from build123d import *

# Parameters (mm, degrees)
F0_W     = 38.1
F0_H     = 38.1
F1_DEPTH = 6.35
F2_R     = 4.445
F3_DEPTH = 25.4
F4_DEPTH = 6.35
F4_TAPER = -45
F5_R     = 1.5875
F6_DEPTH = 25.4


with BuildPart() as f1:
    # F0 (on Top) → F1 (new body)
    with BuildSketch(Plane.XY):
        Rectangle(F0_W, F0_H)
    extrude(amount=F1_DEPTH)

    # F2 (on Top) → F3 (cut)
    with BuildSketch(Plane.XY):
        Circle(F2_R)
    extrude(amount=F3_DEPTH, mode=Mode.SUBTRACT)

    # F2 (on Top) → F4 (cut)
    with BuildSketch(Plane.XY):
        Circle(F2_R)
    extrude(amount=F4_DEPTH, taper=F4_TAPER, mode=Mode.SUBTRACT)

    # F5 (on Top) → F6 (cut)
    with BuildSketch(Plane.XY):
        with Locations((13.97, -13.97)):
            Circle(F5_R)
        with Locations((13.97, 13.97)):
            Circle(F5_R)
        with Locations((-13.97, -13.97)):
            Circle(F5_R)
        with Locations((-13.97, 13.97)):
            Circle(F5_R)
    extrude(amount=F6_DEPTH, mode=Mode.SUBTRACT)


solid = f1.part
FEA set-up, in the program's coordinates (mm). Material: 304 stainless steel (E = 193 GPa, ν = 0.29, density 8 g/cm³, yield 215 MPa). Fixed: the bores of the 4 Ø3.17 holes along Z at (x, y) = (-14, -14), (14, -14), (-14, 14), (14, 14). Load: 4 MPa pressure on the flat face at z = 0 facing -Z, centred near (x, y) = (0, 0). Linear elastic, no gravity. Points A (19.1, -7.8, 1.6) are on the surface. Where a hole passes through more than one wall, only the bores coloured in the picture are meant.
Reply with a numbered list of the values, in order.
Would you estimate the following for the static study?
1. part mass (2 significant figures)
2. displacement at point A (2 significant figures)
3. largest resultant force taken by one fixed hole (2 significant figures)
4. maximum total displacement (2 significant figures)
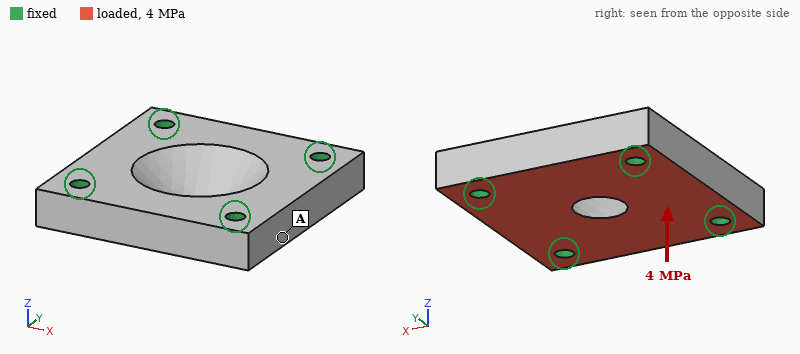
1. 62 g
2. 1.1 µm
3. 1.4 kN
4. 7.0 µm
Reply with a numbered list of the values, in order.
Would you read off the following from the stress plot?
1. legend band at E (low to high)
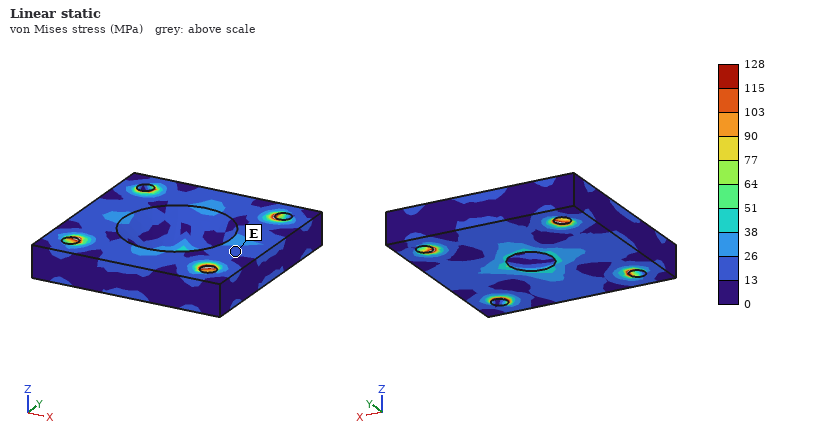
1. 13 to 26 MPa
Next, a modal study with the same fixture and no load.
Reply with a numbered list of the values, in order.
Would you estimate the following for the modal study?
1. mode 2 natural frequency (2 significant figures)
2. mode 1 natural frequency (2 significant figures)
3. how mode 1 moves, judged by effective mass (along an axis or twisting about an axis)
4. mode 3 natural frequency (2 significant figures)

1. 33 kHz
2. 27 kHz
3. along Z
4. 33 kHz
